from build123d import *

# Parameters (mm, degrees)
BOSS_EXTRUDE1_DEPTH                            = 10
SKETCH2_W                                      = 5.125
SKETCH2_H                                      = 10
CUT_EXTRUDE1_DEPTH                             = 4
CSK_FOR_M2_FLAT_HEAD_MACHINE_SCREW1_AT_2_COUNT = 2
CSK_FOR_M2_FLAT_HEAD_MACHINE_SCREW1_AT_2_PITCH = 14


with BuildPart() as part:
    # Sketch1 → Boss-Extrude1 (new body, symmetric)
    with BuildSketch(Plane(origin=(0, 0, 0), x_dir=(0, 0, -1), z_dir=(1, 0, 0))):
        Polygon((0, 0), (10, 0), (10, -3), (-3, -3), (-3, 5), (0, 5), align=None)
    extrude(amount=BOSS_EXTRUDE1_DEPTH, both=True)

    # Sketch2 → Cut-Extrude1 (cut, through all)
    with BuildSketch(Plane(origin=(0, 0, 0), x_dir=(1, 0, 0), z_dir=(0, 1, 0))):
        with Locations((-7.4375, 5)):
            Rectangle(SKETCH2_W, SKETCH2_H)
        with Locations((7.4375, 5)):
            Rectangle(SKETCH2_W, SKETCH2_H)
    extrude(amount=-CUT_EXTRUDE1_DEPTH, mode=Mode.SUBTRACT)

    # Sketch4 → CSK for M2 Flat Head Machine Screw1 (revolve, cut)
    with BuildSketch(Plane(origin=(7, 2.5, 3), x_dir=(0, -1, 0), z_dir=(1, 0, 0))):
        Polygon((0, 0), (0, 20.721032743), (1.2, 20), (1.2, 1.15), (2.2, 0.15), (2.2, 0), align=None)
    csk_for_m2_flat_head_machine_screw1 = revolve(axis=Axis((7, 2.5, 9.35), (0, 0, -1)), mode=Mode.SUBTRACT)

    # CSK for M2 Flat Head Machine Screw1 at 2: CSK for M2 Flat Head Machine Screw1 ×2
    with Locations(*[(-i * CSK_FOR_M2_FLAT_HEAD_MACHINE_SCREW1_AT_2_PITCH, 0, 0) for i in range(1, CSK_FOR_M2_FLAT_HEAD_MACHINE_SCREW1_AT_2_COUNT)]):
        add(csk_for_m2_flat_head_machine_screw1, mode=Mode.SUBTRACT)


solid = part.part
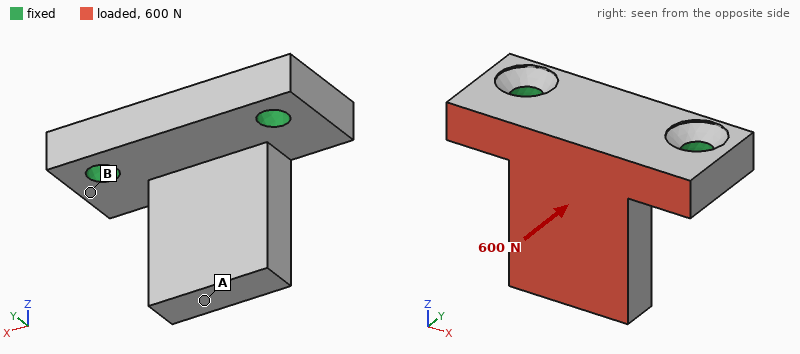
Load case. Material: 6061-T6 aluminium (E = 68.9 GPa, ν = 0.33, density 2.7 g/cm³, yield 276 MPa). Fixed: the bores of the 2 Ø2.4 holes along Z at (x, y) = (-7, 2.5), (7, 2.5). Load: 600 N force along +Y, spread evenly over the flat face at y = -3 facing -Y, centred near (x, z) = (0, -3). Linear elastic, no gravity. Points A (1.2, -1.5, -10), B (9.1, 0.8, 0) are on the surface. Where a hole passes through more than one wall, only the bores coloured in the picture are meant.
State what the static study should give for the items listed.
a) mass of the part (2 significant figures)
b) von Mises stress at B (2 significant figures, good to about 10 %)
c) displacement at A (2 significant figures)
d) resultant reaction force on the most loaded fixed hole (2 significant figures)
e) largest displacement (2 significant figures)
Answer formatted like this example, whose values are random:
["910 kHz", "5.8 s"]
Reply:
["2.0 g", "63 MPa", "0.11 mm", "310 N", "0.11 mm"]
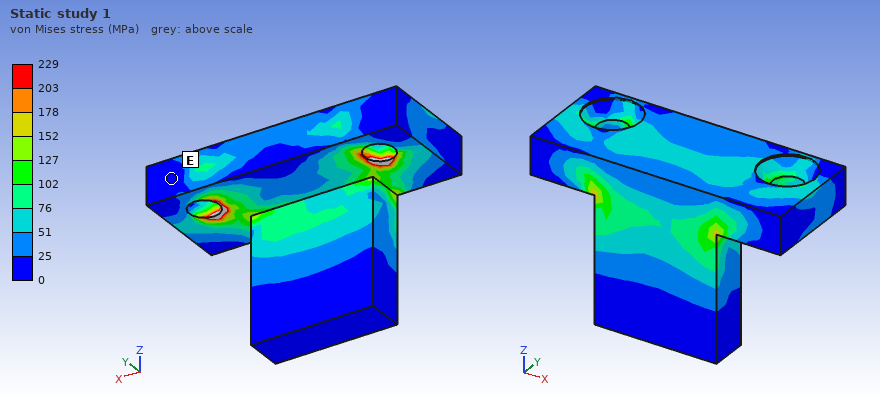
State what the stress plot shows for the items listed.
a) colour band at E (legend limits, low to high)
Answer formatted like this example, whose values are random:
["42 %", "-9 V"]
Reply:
["0 to 25 MPa"]
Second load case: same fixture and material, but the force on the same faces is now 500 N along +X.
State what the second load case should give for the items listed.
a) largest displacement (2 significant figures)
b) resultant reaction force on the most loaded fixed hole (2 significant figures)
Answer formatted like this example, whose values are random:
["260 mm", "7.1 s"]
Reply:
["19 µm", "340 N"]
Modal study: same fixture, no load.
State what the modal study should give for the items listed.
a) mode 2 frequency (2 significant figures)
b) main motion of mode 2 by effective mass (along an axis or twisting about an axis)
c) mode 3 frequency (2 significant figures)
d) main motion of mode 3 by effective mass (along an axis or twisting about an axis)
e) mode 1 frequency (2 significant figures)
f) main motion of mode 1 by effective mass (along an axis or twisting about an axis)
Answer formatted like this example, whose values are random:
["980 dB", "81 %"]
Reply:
["27 kHz", "along X", "34 kHz", "along Z", "12 kHz", "along Y"]
